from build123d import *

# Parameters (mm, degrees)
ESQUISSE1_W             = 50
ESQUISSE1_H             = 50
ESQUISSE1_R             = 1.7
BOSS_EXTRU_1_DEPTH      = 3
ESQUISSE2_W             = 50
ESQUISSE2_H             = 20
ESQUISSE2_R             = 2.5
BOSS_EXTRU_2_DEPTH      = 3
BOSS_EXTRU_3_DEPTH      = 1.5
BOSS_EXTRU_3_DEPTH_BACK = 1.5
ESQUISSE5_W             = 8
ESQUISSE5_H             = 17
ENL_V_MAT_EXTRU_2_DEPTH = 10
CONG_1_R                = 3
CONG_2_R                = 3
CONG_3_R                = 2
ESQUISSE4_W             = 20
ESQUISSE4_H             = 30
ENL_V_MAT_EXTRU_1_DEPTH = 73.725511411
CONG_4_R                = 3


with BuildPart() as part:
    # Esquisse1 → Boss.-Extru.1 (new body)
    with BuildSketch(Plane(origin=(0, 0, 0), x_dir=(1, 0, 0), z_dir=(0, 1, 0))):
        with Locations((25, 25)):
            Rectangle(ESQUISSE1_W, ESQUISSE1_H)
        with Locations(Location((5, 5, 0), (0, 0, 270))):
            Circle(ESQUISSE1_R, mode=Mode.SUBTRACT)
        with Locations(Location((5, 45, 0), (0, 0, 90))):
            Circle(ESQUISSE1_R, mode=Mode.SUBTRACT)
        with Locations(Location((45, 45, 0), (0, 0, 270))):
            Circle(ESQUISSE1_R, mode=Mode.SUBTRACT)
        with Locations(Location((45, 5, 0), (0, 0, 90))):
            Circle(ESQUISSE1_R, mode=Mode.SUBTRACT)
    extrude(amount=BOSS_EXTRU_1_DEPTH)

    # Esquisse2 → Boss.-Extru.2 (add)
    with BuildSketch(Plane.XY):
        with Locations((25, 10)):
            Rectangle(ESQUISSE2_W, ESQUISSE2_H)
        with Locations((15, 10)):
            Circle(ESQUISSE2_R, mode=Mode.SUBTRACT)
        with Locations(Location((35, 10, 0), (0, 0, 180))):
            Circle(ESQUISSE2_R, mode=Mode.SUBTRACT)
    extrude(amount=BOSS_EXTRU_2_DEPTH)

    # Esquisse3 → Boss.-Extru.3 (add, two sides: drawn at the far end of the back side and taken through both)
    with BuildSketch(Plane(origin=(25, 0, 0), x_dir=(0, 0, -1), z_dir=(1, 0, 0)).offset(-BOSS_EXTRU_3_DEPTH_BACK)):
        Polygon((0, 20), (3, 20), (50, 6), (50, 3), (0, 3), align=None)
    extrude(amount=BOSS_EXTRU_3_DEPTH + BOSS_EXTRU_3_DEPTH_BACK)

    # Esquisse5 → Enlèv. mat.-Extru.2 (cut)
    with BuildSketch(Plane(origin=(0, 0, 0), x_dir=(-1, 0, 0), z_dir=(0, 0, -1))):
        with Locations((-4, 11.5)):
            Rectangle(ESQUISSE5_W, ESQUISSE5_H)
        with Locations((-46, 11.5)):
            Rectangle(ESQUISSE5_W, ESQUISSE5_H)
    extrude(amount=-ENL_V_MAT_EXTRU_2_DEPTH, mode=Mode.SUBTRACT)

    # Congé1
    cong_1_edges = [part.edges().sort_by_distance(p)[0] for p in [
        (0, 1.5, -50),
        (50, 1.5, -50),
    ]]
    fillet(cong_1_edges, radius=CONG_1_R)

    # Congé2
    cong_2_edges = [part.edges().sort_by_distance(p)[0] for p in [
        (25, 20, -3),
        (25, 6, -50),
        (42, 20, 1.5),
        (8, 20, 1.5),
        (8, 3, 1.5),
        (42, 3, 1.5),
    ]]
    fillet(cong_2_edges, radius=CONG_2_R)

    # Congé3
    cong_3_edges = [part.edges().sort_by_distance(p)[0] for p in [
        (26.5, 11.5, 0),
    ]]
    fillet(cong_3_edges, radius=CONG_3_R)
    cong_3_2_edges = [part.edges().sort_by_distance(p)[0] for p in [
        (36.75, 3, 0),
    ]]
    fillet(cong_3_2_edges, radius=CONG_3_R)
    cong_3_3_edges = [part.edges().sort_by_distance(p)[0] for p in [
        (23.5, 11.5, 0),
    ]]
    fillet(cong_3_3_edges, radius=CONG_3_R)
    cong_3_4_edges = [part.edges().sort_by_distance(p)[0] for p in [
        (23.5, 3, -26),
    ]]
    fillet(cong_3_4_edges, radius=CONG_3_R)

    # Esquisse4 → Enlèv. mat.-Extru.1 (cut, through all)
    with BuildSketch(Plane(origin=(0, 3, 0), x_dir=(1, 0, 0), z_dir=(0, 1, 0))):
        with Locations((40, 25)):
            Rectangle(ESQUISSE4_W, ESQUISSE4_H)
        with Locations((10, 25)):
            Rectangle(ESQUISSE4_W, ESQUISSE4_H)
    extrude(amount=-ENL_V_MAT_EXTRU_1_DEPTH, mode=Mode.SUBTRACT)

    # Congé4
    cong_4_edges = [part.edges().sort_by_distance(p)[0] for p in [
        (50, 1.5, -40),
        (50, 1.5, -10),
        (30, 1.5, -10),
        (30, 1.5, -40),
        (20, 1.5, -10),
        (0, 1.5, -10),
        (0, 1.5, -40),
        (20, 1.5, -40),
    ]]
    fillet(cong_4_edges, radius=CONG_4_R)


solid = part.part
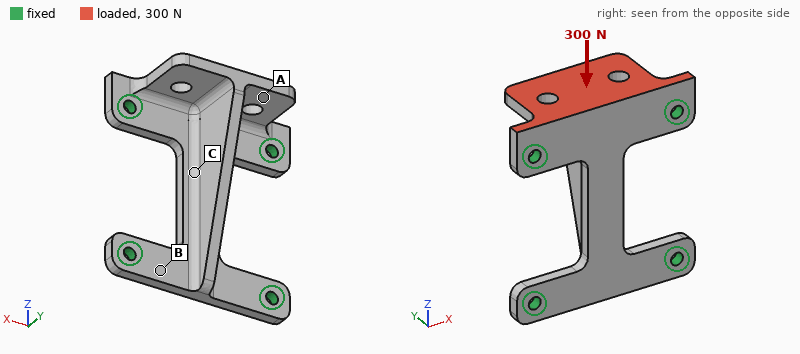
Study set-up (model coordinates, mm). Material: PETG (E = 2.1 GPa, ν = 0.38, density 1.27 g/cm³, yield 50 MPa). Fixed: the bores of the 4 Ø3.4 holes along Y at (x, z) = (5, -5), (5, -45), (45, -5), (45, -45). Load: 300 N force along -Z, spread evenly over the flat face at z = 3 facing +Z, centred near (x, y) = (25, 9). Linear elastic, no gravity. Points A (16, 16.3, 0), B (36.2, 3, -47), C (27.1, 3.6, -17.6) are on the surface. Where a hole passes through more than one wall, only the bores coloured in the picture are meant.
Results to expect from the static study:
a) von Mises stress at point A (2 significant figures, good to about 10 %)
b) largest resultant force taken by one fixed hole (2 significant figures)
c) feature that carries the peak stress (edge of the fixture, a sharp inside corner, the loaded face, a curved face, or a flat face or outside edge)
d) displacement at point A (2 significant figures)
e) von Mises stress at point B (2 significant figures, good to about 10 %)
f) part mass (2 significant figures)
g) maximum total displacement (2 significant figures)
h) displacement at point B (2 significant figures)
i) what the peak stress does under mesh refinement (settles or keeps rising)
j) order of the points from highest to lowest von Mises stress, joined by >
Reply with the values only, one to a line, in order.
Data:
7.4 MPa
110 N
edge of the fixture
0.40 mm
4.2 MPa
9.6 g
0.63 mm
0.11 mm
keeps rising
A > B > C
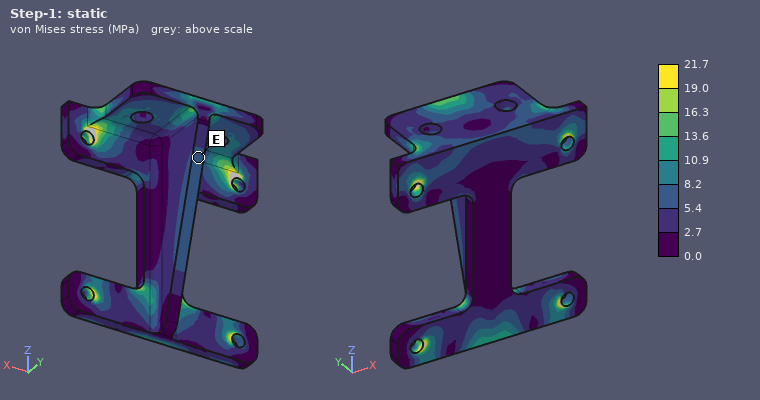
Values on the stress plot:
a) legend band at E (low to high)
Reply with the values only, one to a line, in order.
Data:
5.4 to 8.2 MPa
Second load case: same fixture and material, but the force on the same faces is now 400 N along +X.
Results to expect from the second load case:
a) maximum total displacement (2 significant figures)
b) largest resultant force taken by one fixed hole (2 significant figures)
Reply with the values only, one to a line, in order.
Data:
0.21 mm
230 N
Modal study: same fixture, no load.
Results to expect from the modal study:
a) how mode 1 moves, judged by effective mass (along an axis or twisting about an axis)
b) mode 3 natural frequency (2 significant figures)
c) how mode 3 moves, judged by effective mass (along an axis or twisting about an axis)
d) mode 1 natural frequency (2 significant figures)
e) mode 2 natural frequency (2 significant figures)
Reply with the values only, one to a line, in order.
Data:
along Y
2600 Hz
along X
1600 Hz
2200 Hz
